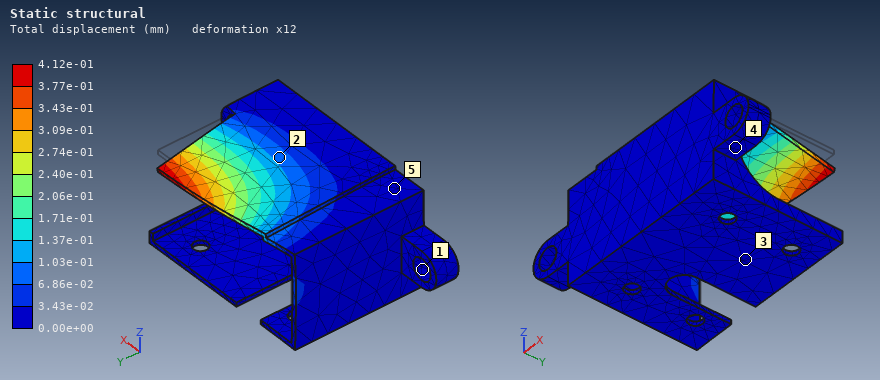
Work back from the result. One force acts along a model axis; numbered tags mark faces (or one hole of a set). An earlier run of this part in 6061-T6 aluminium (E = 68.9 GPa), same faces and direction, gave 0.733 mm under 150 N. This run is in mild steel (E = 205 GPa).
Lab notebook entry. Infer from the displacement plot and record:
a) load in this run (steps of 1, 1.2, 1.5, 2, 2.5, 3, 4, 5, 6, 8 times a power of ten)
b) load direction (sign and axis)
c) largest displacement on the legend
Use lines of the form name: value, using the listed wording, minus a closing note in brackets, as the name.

load in this run: 250 N
load direction: -Z
largest displacement on the legend: 4.12e-01 mm
